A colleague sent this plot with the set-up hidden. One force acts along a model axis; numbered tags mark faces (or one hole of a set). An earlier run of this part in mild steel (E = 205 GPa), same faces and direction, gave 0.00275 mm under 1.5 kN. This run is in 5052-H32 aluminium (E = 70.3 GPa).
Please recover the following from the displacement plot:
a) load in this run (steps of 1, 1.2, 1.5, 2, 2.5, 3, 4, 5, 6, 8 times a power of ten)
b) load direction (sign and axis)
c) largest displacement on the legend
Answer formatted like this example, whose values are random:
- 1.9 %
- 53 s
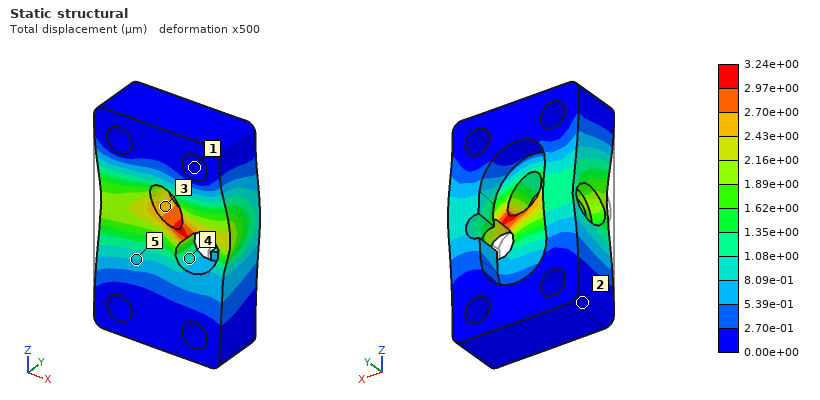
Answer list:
- 600 N
- +X
- 3.24e+00 µm
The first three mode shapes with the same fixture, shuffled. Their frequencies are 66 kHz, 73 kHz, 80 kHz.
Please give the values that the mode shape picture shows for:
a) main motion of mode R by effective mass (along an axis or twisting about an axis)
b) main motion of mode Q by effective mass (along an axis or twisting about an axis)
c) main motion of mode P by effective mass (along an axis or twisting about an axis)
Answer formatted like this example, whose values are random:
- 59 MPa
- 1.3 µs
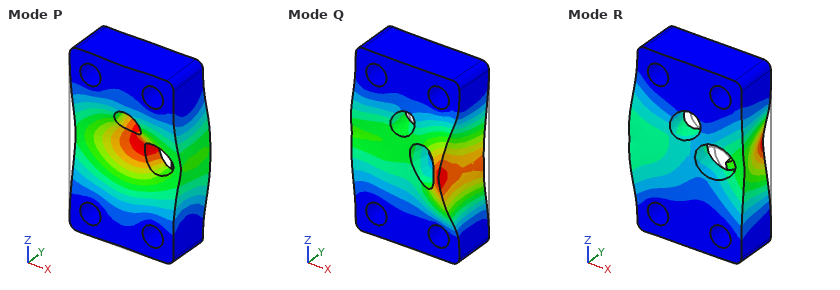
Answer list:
- along X
- along X
- along Y
